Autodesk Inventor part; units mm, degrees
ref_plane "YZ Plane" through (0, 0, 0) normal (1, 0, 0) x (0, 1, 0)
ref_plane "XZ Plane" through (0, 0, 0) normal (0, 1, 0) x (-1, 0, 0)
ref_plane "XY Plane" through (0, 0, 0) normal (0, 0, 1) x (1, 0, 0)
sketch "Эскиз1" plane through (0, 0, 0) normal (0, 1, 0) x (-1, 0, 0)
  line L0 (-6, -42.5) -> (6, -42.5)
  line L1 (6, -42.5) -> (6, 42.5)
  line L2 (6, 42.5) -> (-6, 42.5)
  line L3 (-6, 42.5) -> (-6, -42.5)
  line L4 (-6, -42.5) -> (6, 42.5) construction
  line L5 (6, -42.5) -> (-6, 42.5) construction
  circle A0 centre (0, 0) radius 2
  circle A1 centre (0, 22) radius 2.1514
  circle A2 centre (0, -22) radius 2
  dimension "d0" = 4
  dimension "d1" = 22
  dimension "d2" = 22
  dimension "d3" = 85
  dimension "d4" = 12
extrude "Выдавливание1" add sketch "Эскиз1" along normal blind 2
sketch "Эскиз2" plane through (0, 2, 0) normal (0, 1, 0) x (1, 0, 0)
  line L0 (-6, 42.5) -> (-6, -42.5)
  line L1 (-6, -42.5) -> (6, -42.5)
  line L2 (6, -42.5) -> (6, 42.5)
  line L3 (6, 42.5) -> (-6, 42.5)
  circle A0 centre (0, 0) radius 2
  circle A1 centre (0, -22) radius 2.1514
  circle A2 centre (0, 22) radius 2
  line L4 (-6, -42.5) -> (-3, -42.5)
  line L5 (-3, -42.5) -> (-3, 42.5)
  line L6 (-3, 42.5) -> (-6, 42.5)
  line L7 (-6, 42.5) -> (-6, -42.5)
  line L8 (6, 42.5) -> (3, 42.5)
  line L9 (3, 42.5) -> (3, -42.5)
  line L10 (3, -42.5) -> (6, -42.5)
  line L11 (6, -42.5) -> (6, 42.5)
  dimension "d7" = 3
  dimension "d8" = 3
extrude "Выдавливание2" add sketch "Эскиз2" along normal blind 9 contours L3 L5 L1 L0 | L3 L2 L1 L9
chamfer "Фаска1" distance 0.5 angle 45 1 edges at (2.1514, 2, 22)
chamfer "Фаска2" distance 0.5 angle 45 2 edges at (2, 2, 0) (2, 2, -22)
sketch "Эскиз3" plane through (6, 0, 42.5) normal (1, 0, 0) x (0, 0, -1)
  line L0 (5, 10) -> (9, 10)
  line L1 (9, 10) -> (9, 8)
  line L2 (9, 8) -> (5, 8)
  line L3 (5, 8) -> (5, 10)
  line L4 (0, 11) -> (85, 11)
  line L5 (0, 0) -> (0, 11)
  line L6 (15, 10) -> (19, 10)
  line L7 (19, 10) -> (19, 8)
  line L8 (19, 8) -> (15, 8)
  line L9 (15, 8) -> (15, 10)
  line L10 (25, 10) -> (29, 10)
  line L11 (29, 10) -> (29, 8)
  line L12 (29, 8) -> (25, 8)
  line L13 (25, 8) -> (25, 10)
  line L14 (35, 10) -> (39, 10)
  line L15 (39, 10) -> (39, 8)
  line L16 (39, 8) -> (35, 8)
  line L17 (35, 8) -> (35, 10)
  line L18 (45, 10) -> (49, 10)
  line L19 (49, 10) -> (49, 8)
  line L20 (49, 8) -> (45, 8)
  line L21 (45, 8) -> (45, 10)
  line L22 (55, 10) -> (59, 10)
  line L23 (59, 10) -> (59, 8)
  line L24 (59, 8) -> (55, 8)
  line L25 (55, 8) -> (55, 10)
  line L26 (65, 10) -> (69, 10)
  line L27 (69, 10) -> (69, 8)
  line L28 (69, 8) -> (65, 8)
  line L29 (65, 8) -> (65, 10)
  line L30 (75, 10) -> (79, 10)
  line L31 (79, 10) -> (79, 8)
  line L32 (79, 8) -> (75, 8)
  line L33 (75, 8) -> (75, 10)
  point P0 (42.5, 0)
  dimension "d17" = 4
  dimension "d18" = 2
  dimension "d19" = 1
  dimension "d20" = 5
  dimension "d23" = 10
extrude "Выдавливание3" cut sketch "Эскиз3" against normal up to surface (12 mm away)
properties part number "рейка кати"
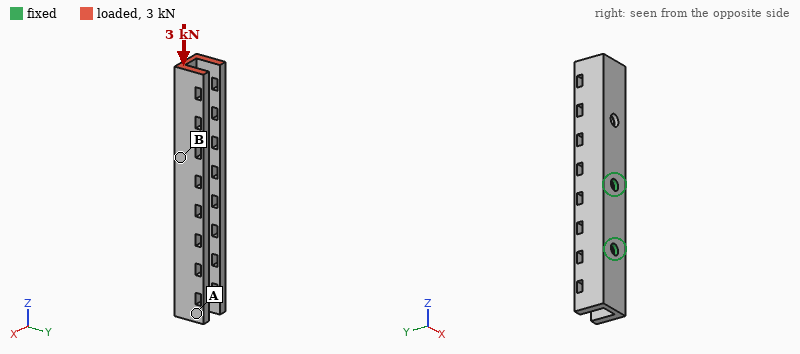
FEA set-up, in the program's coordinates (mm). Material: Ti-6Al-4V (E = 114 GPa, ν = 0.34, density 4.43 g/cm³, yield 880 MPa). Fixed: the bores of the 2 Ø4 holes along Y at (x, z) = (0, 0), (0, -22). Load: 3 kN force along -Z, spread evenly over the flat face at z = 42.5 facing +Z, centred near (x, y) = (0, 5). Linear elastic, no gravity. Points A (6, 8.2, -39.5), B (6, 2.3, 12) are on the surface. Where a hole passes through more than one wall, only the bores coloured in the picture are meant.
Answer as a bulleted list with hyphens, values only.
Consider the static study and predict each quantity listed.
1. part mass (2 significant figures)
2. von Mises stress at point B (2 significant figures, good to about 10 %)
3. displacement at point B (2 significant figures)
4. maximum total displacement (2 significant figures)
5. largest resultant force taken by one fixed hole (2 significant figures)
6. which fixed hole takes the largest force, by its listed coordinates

- 27 g
- 41 MPa
- 17 µm
- 69 µm
- 2.0 kN
- (0, 0)
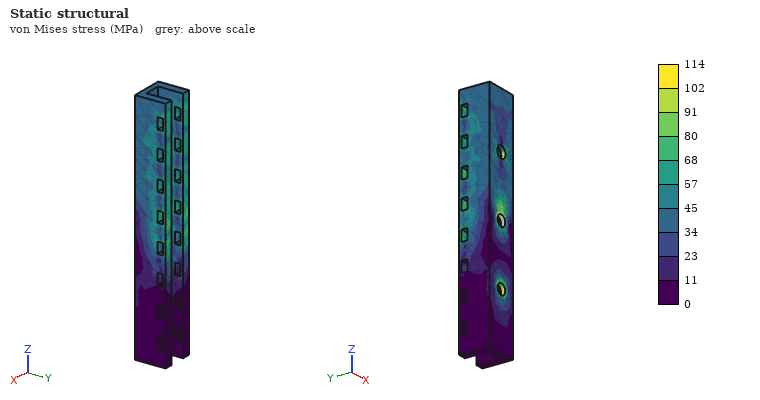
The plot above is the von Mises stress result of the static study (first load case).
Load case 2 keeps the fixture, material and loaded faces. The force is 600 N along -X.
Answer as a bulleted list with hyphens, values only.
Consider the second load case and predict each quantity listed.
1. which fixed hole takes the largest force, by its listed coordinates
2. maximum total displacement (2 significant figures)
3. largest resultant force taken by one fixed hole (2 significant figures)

- (0, 0)
- 0.48 mm
- 1.3 kN
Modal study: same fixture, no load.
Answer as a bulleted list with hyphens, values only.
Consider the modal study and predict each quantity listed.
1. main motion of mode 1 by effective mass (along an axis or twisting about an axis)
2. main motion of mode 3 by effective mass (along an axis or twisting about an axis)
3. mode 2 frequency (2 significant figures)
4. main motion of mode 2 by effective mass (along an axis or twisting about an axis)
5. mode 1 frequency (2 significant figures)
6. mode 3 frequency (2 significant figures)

- along X
- twisting about Z
- 3500 Hz
- along Y
- 3000 Hz
- 6200 Hz
